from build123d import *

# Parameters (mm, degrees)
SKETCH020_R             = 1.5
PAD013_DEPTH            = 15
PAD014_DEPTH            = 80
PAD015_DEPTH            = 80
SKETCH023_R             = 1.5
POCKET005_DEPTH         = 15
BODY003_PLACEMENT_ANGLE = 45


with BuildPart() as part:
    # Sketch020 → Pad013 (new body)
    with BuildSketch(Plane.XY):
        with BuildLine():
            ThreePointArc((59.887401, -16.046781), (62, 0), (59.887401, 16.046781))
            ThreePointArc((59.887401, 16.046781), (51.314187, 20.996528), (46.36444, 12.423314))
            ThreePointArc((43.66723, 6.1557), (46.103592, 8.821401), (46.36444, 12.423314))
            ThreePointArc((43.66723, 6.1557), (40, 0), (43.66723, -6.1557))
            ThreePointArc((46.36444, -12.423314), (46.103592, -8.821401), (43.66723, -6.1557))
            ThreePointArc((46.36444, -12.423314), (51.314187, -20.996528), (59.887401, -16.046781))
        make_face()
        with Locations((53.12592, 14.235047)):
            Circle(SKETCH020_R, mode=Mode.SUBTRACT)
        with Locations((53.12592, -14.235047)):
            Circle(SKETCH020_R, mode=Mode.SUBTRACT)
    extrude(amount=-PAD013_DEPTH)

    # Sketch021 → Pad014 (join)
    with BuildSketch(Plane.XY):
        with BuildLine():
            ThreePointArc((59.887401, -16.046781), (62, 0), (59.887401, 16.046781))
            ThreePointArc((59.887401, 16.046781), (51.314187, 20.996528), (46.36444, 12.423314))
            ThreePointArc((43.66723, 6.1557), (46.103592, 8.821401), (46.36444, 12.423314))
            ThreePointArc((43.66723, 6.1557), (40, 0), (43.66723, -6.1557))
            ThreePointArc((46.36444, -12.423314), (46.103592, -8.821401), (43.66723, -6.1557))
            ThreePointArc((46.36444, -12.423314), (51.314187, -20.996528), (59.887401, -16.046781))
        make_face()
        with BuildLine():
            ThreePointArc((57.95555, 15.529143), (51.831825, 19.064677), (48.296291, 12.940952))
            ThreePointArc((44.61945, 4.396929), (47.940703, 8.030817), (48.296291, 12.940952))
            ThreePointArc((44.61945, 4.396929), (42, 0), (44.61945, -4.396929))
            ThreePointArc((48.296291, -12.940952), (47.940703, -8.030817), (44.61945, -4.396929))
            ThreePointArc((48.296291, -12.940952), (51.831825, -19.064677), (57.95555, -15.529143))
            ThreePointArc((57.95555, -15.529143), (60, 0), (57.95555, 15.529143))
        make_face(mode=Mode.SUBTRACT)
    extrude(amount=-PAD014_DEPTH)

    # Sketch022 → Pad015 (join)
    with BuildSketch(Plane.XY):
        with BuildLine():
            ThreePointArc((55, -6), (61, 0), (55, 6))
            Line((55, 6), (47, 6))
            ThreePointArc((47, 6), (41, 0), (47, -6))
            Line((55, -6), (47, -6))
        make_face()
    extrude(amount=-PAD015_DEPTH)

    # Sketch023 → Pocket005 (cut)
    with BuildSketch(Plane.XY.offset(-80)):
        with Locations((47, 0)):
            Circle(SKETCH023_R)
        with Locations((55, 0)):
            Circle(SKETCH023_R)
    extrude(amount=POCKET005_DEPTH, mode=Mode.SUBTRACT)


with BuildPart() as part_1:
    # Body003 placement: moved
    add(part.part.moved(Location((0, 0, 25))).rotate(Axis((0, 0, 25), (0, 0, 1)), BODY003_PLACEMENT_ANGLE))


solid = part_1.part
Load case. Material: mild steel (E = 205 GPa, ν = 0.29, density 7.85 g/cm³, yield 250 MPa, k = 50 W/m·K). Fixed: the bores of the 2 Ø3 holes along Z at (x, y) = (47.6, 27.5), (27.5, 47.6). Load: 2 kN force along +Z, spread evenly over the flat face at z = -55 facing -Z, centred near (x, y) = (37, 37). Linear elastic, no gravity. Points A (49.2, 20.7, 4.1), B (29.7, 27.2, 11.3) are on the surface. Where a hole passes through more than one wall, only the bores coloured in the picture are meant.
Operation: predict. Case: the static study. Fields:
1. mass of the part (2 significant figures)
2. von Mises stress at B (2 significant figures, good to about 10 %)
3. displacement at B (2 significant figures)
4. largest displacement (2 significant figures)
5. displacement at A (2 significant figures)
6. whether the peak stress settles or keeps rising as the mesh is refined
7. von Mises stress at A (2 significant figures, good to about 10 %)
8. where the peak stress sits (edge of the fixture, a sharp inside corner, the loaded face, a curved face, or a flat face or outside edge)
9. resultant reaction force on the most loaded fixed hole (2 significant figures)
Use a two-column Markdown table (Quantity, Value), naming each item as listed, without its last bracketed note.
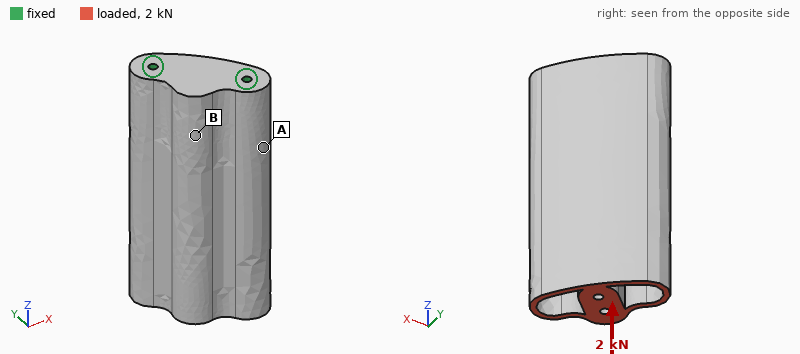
| Quantity | Value |
|---|---|
| mass of the part | 270 g |
| von Mises stress at B | 2.3 MPa |
| displacement at B | 0.93 µm |
| largest displacement | 2.9 µm |
| displacement at A | 0.59 µm |
| whether the peak stress settles or keeps rising as the mesh is refined | keeps rising |
| von Mises stress at A | 7.8 MPa |
| where the peak stress sits | edge of the fixture |
| resultant reaction force on the most loaded fixed hole | 1.0 kN |
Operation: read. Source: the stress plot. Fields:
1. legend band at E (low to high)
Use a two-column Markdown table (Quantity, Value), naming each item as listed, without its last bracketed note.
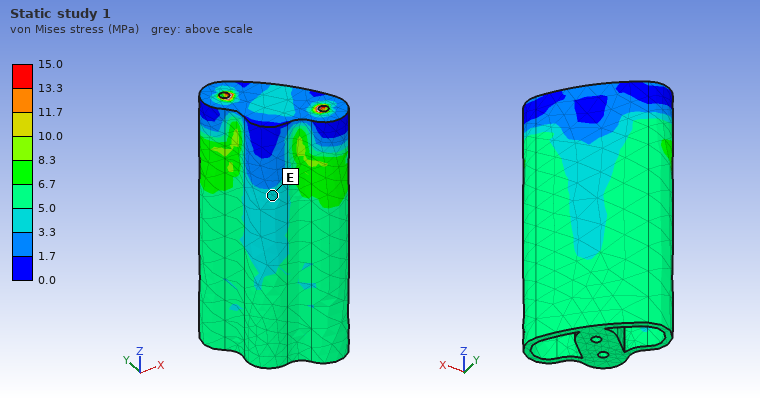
| Quantity | Value |
|---|---|
| legend band at E | 3.3 to 5.0 MPa |
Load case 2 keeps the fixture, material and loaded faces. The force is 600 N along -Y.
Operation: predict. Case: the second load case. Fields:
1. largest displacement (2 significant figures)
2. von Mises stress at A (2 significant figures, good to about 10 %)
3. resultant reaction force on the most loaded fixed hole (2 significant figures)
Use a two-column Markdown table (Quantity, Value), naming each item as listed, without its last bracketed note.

| Quantity | Value |
|---|---|
| largest displacement | 36 µm |
| von Mises stress at A | 25 MPa |
| resultant reaction force on the most loaded fixed hole | 970 N |
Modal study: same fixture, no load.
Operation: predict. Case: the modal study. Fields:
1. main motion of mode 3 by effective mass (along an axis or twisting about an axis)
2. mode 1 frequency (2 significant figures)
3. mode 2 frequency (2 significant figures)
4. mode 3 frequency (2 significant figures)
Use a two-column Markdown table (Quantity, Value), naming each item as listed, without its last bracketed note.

| Quantity | Value |
|---|---|
| main motion of mode 3 by effective mass | twisting about Z |
| mode 1 frequency | 2300 Hz |
| mode 2 frequency | 4400 Hz |
| mode 3 frequency | 8500 Hz |
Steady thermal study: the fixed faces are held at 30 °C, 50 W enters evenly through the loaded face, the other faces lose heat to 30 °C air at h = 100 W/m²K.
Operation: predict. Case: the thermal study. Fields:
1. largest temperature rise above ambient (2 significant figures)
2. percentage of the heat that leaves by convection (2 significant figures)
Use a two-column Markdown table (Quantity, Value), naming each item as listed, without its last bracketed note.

| Quantity | Value |
|---|---|
| largest temperature rise above ambient | 81 K |
| percentage of the heat that leaves by convection | 82 % |
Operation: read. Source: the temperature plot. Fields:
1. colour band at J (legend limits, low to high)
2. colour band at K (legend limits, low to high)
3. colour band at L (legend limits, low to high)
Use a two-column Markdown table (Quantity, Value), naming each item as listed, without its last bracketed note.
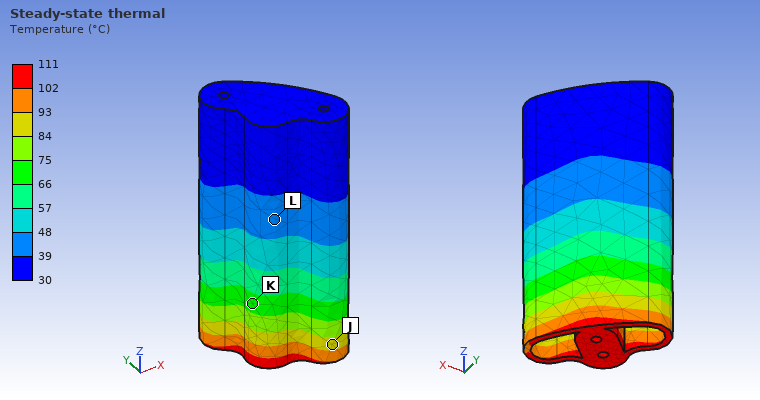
| Quantity | Value |
|---|---|
| colour band at J | 84 to 93 °C |
| colour band at K | 66 to 75 °C |
| colour band at L | 39 to 48 °C |
